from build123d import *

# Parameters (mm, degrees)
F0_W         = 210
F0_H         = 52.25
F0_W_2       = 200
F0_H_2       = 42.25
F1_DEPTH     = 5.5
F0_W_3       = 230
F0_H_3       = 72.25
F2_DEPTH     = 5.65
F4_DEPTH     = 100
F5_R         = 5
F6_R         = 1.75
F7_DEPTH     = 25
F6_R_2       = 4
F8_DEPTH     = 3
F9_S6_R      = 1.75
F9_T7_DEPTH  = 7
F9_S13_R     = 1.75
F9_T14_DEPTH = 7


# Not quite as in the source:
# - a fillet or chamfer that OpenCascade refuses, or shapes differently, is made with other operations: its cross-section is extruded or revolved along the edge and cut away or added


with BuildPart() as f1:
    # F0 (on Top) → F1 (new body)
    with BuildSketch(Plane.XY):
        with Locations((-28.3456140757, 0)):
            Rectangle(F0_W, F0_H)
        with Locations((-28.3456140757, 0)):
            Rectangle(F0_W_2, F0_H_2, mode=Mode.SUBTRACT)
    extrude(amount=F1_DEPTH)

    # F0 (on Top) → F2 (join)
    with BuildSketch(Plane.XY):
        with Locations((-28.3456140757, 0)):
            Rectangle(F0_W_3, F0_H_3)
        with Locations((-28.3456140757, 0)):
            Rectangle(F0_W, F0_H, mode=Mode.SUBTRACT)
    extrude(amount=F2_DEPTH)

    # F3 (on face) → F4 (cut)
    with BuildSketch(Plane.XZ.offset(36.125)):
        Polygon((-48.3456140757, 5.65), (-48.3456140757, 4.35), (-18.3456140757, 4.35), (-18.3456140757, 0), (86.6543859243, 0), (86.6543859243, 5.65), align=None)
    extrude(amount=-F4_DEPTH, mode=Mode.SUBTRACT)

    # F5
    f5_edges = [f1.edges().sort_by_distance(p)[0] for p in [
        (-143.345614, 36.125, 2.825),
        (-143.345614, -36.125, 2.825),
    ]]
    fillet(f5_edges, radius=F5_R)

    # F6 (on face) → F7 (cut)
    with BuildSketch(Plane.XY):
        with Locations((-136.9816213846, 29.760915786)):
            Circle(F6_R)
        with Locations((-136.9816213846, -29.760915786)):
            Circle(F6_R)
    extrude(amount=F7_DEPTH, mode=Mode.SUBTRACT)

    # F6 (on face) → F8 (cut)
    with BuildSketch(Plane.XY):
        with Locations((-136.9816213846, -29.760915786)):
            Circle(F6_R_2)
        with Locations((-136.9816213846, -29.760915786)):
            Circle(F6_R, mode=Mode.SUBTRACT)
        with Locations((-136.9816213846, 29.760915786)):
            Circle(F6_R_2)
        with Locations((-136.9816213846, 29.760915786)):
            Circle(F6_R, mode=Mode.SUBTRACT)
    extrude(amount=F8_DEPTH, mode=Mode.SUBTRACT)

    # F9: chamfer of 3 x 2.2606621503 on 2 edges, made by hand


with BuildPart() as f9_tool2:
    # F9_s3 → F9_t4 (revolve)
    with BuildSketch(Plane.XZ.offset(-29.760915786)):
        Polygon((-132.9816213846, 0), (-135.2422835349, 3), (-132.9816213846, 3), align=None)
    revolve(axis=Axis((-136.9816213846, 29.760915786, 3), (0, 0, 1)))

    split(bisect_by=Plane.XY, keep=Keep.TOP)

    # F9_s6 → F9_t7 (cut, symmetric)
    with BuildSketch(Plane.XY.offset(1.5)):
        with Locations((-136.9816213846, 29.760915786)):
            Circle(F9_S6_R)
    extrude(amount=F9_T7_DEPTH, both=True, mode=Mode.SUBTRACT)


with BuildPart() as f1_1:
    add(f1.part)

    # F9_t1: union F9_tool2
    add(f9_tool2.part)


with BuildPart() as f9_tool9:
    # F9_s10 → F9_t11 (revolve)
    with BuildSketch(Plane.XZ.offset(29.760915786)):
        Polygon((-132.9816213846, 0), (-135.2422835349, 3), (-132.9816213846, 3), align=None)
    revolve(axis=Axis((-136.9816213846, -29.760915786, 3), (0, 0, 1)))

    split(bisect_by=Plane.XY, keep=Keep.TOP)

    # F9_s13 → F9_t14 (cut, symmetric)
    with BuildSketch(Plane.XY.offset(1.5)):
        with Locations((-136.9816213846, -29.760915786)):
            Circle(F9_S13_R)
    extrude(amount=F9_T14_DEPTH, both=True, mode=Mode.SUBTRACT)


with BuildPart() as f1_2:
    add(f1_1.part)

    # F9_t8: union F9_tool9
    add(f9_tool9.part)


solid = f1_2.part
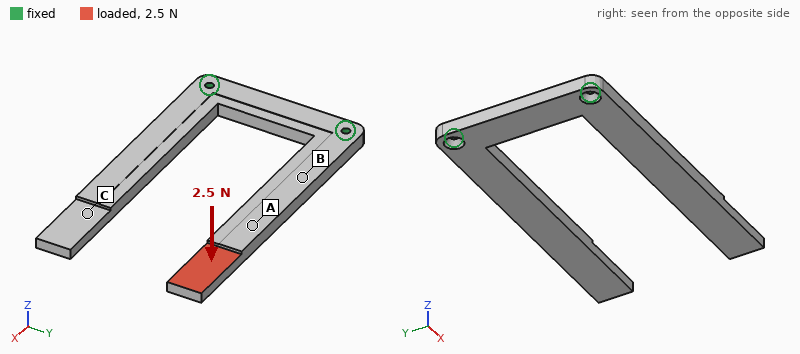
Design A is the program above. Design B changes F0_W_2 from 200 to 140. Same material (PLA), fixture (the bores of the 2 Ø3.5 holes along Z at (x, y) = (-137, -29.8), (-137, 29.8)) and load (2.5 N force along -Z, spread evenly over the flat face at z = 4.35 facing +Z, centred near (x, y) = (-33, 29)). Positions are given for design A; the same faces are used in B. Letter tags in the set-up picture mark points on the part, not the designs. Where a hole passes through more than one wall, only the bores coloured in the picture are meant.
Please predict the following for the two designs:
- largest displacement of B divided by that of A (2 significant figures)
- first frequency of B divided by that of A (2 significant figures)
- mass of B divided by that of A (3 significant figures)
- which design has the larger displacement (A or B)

0.65
1.1
1.30
A
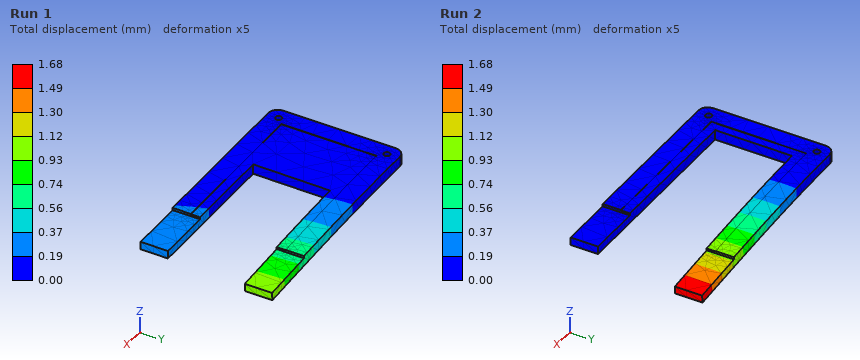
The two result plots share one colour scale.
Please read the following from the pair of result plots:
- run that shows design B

Run 1
